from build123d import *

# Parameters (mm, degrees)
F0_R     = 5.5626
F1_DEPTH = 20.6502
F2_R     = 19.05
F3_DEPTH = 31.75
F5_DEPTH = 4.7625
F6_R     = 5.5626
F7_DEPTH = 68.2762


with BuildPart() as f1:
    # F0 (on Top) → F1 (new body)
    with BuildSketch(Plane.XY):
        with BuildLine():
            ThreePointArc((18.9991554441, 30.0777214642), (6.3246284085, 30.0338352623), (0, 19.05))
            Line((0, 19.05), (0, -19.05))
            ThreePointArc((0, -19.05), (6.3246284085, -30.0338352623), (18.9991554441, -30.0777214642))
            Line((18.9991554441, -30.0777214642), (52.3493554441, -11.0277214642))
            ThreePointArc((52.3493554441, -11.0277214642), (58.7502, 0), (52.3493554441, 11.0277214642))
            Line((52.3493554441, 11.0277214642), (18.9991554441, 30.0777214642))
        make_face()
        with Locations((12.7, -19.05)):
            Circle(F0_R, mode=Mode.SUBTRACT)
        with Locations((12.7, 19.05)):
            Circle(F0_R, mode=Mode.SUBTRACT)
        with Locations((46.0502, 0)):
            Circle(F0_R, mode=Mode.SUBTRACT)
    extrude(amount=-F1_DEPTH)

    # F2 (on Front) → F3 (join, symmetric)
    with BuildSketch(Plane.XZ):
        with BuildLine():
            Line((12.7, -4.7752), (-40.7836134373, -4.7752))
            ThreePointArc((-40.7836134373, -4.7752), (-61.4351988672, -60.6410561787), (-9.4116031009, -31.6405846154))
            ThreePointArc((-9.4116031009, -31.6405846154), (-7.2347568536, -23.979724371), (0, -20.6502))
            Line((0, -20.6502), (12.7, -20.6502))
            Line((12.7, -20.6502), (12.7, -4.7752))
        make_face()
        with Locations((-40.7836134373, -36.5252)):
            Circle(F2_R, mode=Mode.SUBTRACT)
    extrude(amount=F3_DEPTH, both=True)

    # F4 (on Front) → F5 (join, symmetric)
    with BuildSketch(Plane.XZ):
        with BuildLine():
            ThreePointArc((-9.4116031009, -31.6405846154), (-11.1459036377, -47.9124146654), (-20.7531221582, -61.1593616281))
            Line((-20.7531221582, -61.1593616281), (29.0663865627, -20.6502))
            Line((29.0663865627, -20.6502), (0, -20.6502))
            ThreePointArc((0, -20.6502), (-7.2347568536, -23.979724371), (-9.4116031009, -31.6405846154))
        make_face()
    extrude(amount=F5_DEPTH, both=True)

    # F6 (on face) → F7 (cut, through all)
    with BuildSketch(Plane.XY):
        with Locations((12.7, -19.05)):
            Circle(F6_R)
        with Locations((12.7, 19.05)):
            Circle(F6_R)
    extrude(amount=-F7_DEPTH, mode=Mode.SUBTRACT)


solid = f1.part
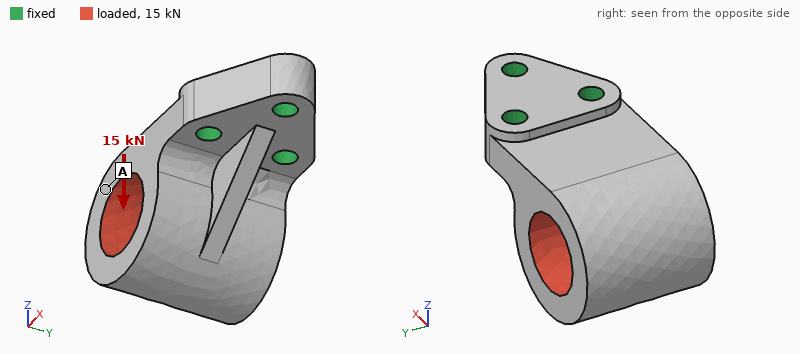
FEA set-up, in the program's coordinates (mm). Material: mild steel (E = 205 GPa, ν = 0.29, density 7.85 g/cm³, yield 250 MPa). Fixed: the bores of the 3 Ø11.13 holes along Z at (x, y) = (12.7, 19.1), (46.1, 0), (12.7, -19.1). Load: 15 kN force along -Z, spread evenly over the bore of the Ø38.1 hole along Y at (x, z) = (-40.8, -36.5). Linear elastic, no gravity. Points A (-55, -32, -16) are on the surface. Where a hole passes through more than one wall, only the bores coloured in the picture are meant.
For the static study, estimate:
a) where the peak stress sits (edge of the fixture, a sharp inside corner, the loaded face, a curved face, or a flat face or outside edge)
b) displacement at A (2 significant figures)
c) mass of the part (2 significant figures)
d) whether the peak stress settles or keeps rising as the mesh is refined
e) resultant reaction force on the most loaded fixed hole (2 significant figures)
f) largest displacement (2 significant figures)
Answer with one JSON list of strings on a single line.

["edge of the fixture", "0.10 mm", "1.6 kg", "keeps rising", "11 kN", "0.14 mm"]
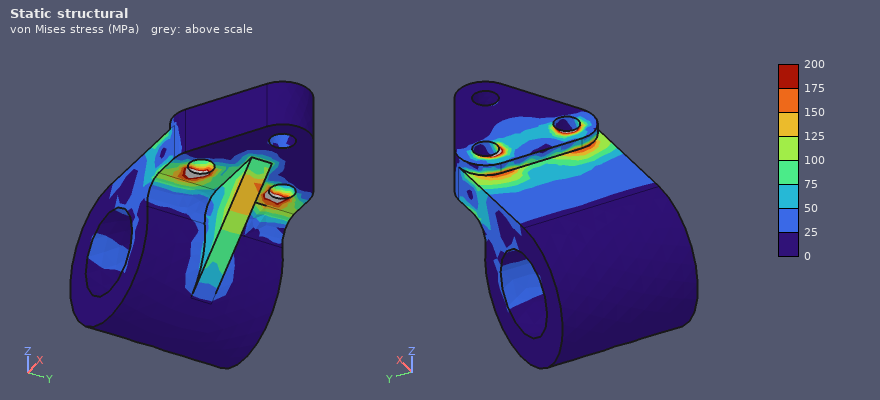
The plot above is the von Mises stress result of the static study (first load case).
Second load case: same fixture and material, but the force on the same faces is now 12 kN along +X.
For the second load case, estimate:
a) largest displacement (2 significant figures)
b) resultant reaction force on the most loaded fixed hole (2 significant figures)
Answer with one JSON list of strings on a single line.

["62 µm", "4.9 kN"]
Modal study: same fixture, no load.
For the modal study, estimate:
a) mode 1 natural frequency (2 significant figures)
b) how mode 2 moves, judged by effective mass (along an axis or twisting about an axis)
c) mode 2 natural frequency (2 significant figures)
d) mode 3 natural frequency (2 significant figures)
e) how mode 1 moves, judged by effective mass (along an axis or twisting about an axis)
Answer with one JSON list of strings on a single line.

["1700 Hz", "along Y", "3200 Hz", "5200 Hz", "along Z"]
